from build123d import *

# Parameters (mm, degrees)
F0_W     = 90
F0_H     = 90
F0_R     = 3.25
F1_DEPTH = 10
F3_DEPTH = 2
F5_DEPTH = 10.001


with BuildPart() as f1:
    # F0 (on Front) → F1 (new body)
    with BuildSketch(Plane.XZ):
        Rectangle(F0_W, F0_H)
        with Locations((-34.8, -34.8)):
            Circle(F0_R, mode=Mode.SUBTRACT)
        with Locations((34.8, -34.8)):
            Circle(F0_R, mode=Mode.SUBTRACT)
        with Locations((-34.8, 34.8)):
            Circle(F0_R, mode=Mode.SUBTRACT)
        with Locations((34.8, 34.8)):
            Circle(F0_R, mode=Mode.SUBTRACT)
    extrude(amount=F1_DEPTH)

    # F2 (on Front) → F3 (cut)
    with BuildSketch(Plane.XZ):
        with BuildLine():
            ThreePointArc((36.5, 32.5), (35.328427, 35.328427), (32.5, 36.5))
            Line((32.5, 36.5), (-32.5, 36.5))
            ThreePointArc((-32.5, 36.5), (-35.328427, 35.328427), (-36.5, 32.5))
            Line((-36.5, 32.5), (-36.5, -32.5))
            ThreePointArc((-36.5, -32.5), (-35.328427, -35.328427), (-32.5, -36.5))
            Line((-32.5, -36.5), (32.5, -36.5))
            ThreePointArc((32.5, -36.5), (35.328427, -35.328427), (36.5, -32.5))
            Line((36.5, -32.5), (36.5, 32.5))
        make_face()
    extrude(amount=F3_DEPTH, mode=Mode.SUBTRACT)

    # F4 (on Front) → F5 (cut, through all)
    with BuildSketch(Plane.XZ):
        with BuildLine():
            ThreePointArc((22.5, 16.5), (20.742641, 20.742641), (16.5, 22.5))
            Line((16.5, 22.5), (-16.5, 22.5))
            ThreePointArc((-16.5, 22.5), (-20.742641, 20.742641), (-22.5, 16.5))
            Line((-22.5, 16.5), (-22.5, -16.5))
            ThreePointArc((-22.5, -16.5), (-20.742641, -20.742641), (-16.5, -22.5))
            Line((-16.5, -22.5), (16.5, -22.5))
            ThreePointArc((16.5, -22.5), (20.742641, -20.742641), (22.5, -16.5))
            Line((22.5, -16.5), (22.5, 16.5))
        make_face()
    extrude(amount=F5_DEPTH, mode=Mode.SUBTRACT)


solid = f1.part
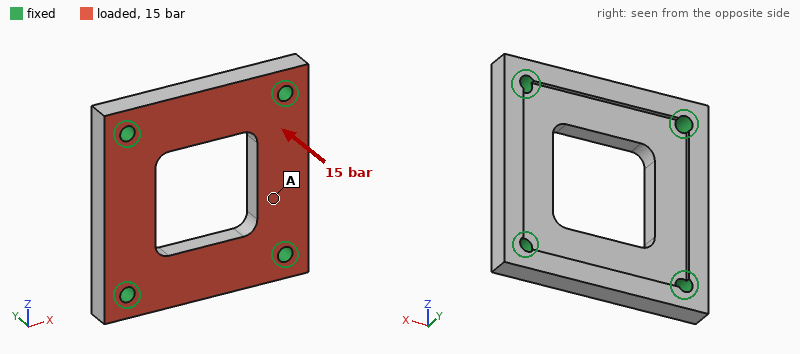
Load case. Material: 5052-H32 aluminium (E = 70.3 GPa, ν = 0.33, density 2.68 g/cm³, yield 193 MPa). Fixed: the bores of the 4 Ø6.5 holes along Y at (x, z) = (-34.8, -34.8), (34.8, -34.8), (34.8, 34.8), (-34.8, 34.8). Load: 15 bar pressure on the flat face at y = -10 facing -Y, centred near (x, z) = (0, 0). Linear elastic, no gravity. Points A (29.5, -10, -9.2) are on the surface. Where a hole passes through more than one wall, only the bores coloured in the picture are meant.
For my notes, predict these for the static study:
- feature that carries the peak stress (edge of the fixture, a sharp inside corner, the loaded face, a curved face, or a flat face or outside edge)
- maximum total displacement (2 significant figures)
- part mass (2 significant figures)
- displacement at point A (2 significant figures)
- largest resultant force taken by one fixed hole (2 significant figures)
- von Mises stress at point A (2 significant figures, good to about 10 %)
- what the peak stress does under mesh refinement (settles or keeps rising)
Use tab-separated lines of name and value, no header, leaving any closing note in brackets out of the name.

feature that carries the peak stress	edge of the fixture
maximum total displacement	37 µm
part mass	140 g
displacement at point A	27 µm
largest resultant force taken by one fixed hole	2.2 kN
von Mises stress at point A	17 MPa
what the peak stress does under mesh refinement	keeps rising
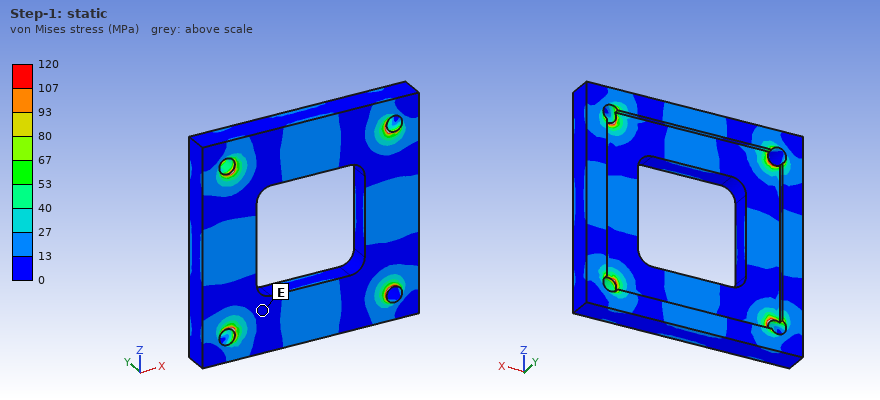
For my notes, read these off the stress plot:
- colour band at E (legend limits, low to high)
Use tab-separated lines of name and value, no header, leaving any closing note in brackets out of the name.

colour band at E	0 to 13 MPa
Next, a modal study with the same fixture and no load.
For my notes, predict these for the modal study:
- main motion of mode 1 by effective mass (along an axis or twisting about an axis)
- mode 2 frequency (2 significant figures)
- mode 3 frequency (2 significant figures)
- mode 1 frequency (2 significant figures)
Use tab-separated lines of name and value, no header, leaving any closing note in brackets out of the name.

main motion of mode 1 by effective mass	along Y
mode 2 frequency	9400 Hz
mode 3 frequency	9400 Hz
mode 1 frequency	8500 Hz
